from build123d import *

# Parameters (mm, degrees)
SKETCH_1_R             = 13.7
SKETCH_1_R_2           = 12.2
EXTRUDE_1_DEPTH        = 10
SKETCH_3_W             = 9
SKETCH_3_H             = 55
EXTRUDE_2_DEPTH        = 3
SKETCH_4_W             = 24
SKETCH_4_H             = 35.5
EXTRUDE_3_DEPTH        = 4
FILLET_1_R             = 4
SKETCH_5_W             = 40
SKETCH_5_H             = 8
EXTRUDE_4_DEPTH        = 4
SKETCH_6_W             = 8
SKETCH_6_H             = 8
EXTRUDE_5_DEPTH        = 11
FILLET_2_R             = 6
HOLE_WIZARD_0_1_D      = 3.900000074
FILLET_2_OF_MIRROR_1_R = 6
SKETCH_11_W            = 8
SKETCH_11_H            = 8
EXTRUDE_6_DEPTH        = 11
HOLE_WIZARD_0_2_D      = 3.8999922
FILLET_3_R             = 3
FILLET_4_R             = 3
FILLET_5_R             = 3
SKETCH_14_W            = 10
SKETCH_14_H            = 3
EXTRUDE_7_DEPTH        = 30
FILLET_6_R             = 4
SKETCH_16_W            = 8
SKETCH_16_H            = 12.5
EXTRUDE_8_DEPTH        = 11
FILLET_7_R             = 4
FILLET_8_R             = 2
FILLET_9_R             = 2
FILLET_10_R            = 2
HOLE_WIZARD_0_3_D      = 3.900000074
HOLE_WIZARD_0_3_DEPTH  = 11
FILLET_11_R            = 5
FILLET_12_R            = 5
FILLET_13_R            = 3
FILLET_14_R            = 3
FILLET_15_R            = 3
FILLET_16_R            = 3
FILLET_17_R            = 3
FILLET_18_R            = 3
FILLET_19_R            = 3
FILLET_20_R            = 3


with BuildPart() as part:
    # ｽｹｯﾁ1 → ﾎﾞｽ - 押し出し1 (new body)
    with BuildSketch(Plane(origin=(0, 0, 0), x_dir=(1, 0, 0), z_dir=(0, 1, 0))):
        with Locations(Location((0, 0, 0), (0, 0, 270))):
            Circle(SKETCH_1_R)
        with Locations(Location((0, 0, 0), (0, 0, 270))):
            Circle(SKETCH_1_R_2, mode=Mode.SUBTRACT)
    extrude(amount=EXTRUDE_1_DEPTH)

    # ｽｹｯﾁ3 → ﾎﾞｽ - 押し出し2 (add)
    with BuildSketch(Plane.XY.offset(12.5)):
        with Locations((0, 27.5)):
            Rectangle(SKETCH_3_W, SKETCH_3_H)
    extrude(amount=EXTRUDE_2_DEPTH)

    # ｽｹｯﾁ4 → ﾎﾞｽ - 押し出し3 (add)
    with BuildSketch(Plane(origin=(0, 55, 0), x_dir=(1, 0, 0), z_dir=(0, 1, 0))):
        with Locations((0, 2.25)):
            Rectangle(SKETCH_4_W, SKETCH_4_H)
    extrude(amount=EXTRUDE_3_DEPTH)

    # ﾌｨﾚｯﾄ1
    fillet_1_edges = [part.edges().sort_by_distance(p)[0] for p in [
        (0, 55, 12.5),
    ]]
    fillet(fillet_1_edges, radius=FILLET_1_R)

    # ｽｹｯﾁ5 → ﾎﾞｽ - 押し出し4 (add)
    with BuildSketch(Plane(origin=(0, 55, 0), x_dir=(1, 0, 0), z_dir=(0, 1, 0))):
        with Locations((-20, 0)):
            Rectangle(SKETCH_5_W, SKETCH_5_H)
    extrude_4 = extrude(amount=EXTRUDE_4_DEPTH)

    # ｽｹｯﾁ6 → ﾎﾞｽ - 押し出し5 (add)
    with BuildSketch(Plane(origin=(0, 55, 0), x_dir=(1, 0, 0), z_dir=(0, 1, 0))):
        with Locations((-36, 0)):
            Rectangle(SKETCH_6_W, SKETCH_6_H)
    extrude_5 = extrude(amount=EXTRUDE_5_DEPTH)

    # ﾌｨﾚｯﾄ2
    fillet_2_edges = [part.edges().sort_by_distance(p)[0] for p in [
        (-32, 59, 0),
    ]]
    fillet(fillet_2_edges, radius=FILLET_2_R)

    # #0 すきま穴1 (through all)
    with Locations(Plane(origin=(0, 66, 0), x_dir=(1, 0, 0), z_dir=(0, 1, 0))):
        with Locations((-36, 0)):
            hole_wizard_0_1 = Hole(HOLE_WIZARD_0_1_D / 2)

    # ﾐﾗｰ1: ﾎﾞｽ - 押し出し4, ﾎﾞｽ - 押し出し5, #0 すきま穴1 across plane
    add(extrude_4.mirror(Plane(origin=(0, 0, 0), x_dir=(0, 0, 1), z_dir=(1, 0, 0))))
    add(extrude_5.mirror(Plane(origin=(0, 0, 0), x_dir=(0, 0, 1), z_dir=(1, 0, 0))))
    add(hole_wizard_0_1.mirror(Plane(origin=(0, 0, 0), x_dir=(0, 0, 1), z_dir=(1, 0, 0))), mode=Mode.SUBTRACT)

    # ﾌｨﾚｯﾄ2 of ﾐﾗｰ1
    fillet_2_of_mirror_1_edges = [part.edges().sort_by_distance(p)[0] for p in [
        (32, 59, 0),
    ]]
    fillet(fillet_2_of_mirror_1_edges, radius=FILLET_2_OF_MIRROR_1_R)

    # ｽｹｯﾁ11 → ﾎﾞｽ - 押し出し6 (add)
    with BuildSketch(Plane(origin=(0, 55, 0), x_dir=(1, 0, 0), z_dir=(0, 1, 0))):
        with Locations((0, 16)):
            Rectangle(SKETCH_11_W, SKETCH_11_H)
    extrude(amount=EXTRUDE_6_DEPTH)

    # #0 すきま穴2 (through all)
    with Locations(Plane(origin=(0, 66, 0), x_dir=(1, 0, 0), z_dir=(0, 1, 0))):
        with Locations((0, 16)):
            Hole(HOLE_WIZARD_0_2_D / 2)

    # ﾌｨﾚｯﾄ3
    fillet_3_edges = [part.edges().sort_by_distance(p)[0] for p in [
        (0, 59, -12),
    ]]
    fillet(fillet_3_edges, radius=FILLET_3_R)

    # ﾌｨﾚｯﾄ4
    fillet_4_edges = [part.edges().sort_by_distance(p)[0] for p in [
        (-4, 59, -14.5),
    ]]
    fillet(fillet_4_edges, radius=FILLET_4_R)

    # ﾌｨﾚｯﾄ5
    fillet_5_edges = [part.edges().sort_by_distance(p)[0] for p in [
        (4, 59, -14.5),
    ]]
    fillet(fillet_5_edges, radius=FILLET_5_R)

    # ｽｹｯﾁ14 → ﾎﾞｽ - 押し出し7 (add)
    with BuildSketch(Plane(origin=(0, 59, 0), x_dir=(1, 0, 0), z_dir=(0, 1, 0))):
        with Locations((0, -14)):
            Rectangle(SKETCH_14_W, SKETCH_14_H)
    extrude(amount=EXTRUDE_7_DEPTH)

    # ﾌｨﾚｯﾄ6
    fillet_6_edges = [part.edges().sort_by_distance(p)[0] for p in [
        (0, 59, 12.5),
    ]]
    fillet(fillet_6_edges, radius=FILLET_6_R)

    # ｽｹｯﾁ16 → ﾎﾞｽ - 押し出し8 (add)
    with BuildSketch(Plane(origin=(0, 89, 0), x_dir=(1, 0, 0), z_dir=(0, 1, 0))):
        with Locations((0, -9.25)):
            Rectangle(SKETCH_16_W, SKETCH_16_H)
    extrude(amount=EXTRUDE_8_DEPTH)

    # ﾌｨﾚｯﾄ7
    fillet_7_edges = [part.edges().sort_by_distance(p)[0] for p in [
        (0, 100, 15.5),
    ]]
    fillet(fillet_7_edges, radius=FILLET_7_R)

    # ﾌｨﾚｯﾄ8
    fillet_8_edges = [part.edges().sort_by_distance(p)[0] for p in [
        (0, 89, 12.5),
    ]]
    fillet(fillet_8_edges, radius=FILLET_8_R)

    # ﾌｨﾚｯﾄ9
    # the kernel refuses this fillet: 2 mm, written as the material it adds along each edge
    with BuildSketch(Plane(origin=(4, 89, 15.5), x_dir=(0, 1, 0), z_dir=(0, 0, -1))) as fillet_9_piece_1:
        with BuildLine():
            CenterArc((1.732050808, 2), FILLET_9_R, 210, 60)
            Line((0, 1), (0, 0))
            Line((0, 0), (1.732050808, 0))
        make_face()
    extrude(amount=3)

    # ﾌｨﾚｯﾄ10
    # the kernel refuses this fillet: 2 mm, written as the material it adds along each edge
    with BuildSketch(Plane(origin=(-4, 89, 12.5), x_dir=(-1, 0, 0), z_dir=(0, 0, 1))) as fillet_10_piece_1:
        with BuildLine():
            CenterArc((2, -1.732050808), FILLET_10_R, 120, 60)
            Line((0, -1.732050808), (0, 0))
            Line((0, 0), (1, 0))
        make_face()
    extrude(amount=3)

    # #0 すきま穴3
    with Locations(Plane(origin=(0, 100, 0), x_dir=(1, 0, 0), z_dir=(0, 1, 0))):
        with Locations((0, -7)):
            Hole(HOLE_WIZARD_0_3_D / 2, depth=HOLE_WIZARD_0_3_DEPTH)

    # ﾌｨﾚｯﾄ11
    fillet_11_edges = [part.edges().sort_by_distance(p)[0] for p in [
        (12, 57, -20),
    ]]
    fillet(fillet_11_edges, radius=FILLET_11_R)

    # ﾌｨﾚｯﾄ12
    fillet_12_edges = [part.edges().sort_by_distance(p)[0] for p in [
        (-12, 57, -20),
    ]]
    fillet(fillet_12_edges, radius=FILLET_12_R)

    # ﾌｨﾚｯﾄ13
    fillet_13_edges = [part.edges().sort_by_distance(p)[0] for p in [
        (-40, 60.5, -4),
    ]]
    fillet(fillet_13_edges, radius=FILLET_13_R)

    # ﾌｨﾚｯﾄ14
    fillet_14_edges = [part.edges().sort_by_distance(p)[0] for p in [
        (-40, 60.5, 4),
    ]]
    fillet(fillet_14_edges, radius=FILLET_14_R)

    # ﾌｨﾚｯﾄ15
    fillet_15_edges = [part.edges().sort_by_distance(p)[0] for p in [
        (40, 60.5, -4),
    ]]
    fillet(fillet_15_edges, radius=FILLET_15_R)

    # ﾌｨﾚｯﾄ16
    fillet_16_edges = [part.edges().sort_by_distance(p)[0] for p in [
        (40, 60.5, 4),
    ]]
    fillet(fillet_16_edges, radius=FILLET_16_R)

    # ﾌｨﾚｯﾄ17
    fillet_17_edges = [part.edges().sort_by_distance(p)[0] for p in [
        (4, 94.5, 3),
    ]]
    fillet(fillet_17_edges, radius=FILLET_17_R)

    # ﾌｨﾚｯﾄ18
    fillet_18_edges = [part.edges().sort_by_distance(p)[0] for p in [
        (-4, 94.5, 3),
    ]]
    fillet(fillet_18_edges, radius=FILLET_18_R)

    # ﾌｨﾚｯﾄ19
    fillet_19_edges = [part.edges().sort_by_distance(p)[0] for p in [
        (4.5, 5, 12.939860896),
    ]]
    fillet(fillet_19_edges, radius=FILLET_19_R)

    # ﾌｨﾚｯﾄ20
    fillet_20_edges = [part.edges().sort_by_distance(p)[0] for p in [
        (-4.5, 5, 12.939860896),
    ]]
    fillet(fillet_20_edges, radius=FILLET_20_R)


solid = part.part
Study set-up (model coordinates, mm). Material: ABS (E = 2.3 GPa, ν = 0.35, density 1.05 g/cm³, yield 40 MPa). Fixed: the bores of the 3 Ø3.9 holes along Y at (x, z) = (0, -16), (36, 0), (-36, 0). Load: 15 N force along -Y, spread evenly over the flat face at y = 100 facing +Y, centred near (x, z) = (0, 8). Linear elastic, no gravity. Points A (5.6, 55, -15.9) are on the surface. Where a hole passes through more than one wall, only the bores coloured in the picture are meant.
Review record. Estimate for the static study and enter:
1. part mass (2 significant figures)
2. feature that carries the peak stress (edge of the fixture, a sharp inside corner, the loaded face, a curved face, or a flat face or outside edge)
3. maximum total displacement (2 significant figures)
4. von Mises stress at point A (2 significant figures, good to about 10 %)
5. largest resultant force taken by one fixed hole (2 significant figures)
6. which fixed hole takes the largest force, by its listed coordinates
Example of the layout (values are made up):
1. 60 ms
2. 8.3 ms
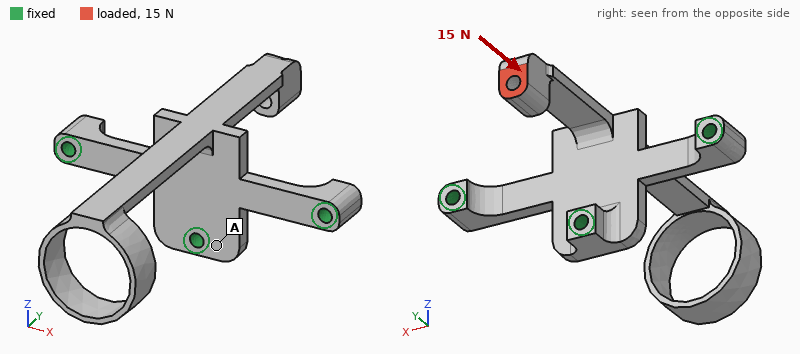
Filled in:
1. 11 g
2. a curved face
3. 1.3 mm
4. 0.88 MPa
5. 9.1 N
6. (0, -16)
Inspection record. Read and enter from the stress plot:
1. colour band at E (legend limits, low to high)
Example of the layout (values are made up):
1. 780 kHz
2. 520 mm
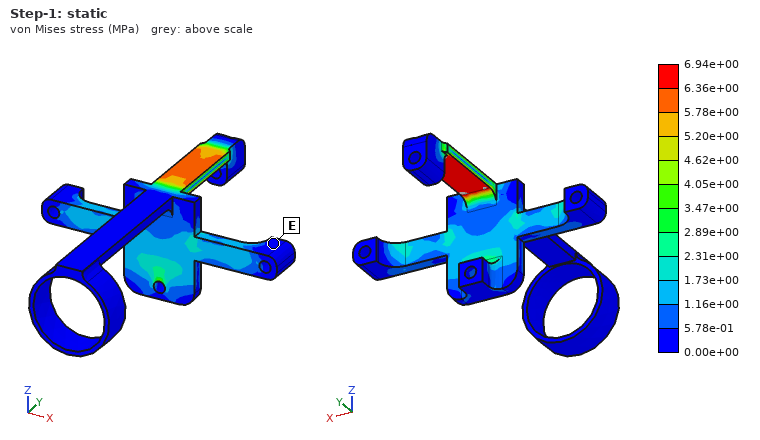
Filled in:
1. 0.00e+00 to 5.78e-01 MPa
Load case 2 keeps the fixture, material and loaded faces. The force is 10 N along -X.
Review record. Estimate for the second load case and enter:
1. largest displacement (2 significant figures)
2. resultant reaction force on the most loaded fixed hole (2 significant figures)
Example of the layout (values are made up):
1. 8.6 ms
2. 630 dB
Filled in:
1. 1.4 mm
2. 8.6 N
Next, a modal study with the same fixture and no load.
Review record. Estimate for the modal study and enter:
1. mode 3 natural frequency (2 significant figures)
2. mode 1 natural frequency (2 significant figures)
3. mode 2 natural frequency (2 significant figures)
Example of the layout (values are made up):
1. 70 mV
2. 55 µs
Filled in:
1. 250 Hz
2. 110 Hz
3. 190 Hz
